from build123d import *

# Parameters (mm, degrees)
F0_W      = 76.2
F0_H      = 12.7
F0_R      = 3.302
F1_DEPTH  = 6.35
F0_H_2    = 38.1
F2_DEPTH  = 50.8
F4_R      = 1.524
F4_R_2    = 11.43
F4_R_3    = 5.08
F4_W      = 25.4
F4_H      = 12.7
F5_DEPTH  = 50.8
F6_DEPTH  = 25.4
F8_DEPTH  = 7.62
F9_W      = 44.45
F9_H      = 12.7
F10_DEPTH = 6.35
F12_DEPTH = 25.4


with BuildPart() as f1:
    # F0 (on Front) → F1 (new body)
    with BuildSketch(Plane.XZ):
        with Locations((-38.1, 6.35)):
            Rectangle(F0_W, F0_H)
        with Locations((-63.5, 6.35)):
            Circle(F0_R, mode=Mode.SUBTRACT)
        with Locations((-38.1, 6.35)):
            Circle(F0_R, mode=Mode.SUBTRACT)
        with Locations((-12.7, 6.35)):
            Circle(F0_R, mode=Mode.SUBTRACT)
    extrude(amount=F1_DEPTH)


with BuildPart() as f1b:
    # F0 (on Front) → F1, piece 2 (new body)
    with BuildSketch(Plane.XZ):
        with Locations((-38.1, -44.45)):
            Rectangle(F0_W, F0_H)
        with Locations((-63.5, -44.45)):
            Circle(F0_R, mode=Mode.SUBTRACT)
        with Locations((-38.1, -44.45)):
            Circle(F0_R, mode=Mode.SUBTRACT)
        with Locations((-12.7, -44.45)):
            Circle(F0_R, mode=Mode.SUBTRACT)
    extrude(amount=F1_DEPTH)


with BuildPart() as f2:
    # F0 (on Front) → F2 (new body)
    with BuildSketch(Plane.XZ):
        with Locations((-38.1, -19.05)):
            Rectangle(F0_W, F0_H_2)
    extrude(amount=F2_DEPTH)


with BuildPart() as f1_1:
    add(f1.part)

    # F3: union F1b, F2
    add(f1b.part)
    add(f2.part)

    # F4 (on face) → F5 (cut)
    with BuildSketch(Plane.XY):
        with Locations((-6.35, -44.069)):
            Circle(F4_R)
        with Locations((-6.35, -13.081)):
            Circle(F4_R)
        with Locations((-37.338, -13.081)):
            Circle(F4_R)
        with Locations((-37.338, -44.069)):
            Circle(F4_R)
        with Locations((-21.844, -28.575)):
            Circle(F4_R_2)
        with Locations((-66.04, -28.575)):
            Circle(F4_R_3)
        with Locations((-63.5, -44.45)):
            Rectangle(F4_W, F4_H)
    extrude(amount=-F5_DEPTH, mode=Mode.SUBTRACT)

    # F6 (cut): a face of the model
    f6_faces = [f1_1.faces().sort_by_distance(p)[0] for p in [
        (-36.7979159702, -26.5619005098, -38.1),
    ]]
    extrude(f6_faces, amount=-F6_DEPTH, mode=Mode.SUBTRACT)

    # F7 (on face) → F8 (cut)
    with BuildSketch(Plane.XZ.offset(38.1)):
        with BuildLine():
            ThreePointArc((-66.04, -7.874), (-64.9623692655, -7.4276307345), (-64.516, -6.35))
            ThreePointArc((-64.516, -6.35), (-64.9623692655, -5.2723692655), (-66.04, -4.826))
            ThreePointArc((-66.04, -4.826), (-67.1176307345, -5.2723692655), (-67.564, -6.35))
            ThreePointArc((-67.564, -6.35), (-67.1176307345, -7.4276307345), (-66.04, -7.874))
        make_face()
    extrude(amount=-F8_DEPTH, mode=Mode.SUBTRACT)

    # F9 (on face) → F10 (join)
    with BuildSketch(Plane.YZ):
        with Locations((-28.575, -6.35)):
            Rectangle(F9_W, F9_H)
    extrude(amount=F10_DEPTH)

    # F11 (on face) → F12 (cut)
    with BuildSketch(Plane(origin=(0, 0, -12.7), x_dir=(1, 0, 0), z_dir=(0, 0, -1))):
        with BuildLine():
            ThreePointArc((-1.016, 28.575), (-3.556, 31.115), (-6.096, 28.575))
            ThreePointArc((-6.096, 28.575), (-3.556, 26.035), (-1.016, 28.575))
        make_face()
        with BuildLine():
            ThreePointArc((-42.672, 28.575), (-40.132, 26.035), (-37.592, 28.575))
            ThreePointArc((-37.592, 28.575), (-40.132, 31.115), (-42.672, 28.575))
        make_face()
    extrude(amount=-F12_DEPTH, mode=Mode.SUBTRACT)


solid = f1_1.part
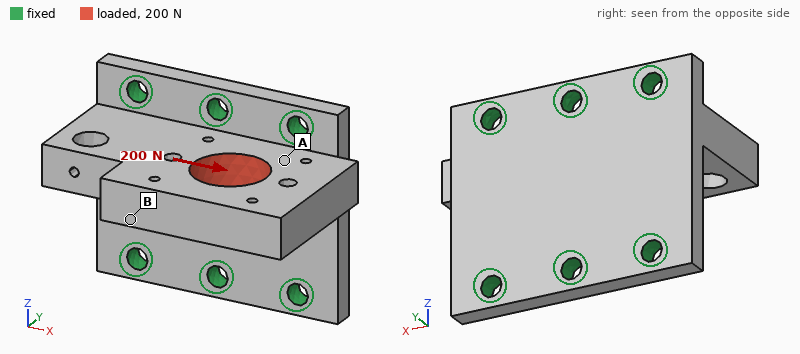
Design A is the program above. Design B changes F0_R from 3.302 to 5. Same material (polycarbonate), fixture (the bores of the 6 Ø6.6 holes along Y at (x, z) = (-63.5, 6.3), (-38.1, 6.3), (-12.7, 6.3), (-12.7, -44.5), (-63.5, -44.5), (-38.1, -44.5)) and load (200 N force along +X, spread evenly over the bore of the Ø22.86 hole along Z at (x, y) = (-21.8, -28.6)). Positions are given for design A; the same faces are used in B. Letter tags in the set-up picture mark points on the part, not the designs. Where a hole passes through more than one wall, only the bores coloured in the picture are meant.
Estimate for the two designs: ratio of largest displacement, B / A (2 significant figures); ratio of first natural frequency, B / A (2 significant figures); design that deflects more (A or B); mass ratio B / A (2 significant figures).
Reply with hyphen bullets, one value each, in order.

- 0.79
- 1.1
- A
- 0.97
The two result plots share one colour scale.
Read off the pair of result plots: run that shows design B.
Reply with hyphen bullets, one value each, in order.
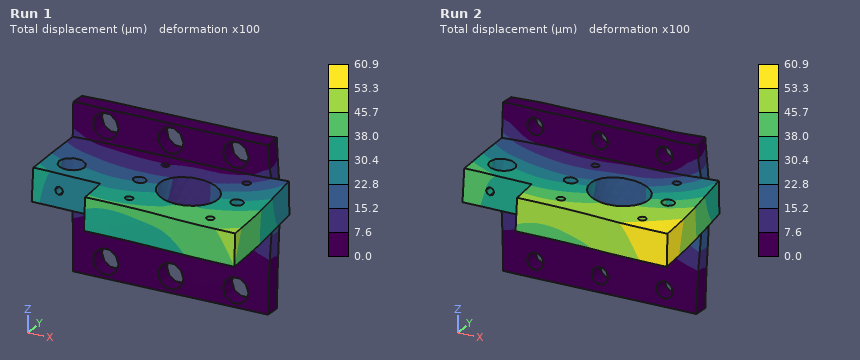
- Run 1
